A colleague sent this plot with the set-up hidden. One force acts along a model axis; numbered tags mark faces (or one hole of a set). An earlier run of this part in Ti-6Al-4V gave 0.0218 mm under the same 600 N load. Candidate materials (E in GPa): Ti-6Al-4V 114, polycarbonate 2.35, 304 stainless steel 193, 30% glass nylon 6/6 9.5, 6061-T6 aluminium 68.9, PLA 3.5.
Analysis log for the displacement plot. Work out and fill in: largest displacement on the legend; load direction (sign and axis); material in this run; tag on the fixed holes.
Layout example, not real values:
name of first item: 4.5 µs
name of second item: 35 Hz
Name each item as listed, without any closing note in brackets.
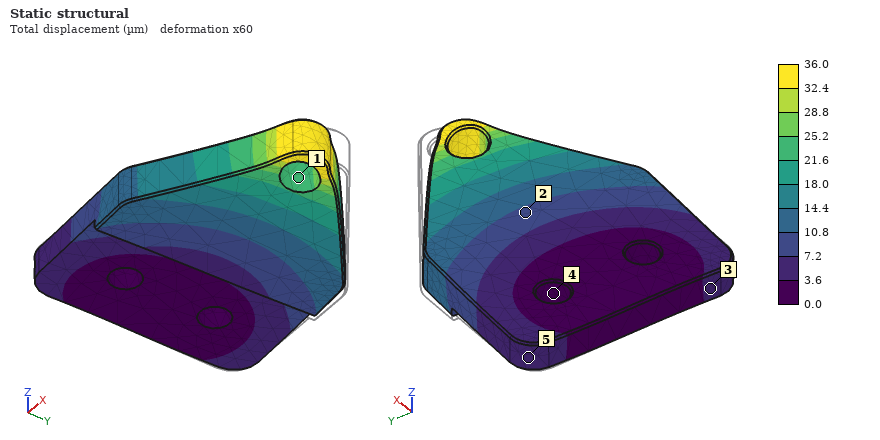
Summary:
largest displacement on the legend: 36.0 µm
load direction: -Y
material in this run: 6061-T6 aluminium
tag on the fixed holes: 4
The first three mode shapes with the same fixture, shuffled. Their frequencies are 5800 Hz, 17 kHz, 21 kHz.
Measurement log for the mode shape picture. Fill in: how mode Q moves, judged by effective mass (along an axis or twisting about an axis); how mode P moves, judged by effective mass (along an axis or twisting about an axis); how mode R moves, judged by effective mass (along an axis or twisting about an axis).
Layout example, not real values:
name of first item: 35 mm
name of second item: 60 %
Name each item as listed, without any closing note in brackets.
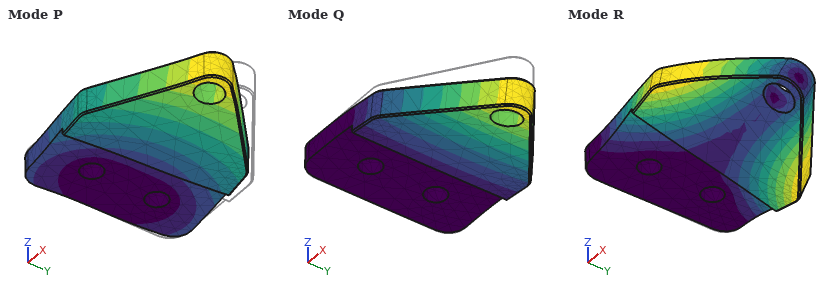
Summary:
how mode Q moves, judged by effective mass: along Z
how mode P moves, judged by effective mass: along Y
how mode R moves, judged by effective mass: twisting about X
